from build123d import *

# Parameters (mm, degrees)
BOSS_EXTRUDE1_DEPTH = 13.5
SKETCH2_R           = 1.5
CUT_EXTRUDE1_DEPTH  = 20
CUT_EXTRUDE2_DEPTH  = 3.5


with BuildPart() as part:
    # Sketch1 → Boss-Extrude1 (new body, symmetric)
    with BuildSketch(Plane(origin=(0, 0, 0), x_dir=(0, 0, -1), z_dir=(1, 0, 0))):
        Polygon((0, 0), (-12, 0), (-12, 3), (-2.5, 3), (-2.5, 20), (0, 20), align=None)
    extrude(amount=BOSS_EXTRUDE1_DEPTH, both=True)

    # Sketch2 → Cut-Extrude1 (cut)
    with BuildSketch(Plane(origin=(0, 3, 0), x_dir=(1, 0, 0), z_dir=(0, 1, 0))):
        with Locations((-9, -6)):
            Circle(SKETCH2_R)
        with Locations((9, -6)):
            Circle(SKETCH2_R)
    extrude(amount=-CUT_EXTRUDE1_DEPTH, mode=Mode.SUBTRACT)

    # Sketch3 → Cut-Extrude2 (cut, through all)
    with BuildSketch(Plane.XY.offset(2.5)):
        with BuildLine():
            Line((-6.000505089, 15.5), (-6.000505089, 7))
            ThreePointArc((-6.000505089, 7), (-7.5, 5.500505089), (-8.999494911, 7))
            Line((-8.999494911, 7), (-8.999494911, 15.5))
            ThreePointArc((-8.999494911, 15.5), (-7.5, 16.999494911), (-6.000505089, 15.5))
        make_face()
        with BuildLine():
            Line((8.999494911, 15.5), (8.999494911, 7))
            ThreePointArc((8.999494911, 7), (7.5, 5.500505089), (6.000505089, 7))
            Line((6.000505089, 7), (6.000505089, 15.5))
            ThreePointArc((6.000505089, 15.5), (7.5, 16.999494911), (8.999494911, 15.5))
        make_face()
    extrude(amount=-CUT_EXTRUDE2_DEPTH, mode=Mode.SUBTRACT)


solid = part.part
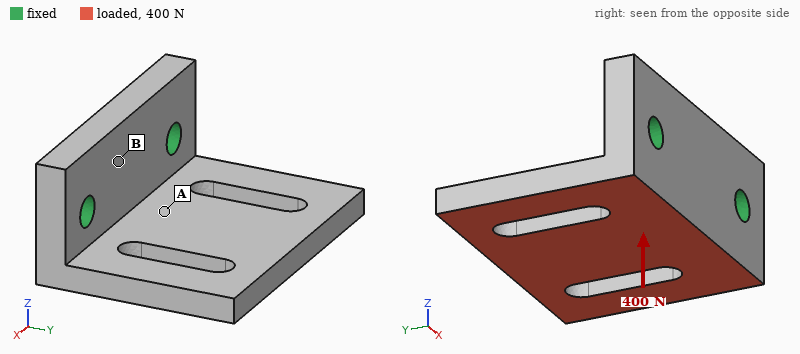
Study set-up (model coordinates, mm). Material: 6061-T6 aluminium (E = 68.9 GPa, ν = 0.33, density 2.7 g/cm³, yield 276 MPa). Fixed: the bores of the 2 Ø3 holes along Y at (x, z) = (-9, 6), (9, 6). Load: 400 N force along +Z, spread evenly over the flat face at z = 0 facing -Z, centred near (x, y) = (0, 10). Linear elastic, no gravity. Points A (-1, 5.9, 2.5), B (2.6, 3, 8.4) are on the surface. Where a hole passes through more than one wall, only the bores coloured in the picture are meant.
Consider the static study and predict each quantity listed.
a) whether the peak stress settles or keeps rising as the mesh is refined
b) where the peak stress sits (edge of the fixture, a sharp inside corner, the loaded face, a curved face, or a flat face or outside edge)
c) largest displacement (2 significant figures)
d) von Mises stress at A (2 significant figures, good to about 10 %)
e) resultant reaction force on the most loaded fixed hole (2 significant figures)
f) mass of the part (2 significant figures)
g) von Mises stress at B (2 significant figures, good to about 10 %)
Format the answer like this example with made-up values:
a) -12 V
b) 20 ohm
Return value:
a) keeps rising
b) edge of the fixture
c) 0.18 mm
d) 77 MPa
e) 200 N
f) 5.2 g
g) 17 MPa
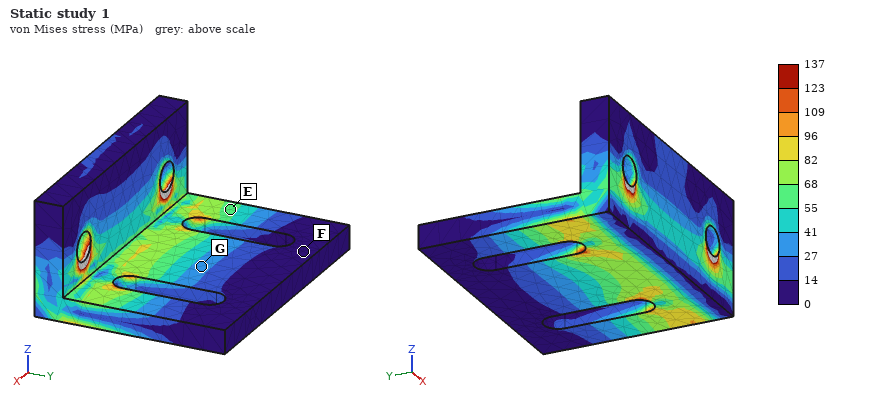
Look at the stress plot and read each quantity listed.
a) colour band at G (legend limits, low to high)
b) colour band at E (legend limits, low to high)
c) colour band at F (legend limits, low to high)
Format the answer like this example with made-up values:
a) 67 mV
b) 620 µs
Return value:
a) 27 to 41 MPa
b) 55 to 68 MPa
c) 0 to 14 MPa
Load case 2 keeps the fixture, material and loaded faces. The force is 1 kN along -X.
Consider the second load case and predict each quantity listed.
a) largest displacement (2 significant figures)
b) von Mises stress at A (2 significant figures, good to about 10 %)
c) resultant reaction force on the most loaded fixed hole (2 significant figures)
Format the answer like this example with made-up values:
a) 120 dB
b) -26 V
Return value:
a) 36 µm
b) 19 MPa
c) 710 N
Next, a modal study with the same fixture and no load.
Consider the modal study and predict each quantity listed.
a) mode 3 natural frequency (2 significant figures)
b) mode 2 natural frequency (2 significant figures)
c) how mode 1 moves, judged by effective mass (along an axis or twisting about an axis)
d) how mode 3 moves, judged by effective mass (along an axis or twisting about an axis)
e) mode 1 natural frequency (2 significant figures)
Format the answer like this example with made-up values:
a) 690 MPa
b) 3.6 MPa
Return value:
a) 18 kHz
b) 9500 Hz
c) along Z
d) along X
e) 5100 Hz
